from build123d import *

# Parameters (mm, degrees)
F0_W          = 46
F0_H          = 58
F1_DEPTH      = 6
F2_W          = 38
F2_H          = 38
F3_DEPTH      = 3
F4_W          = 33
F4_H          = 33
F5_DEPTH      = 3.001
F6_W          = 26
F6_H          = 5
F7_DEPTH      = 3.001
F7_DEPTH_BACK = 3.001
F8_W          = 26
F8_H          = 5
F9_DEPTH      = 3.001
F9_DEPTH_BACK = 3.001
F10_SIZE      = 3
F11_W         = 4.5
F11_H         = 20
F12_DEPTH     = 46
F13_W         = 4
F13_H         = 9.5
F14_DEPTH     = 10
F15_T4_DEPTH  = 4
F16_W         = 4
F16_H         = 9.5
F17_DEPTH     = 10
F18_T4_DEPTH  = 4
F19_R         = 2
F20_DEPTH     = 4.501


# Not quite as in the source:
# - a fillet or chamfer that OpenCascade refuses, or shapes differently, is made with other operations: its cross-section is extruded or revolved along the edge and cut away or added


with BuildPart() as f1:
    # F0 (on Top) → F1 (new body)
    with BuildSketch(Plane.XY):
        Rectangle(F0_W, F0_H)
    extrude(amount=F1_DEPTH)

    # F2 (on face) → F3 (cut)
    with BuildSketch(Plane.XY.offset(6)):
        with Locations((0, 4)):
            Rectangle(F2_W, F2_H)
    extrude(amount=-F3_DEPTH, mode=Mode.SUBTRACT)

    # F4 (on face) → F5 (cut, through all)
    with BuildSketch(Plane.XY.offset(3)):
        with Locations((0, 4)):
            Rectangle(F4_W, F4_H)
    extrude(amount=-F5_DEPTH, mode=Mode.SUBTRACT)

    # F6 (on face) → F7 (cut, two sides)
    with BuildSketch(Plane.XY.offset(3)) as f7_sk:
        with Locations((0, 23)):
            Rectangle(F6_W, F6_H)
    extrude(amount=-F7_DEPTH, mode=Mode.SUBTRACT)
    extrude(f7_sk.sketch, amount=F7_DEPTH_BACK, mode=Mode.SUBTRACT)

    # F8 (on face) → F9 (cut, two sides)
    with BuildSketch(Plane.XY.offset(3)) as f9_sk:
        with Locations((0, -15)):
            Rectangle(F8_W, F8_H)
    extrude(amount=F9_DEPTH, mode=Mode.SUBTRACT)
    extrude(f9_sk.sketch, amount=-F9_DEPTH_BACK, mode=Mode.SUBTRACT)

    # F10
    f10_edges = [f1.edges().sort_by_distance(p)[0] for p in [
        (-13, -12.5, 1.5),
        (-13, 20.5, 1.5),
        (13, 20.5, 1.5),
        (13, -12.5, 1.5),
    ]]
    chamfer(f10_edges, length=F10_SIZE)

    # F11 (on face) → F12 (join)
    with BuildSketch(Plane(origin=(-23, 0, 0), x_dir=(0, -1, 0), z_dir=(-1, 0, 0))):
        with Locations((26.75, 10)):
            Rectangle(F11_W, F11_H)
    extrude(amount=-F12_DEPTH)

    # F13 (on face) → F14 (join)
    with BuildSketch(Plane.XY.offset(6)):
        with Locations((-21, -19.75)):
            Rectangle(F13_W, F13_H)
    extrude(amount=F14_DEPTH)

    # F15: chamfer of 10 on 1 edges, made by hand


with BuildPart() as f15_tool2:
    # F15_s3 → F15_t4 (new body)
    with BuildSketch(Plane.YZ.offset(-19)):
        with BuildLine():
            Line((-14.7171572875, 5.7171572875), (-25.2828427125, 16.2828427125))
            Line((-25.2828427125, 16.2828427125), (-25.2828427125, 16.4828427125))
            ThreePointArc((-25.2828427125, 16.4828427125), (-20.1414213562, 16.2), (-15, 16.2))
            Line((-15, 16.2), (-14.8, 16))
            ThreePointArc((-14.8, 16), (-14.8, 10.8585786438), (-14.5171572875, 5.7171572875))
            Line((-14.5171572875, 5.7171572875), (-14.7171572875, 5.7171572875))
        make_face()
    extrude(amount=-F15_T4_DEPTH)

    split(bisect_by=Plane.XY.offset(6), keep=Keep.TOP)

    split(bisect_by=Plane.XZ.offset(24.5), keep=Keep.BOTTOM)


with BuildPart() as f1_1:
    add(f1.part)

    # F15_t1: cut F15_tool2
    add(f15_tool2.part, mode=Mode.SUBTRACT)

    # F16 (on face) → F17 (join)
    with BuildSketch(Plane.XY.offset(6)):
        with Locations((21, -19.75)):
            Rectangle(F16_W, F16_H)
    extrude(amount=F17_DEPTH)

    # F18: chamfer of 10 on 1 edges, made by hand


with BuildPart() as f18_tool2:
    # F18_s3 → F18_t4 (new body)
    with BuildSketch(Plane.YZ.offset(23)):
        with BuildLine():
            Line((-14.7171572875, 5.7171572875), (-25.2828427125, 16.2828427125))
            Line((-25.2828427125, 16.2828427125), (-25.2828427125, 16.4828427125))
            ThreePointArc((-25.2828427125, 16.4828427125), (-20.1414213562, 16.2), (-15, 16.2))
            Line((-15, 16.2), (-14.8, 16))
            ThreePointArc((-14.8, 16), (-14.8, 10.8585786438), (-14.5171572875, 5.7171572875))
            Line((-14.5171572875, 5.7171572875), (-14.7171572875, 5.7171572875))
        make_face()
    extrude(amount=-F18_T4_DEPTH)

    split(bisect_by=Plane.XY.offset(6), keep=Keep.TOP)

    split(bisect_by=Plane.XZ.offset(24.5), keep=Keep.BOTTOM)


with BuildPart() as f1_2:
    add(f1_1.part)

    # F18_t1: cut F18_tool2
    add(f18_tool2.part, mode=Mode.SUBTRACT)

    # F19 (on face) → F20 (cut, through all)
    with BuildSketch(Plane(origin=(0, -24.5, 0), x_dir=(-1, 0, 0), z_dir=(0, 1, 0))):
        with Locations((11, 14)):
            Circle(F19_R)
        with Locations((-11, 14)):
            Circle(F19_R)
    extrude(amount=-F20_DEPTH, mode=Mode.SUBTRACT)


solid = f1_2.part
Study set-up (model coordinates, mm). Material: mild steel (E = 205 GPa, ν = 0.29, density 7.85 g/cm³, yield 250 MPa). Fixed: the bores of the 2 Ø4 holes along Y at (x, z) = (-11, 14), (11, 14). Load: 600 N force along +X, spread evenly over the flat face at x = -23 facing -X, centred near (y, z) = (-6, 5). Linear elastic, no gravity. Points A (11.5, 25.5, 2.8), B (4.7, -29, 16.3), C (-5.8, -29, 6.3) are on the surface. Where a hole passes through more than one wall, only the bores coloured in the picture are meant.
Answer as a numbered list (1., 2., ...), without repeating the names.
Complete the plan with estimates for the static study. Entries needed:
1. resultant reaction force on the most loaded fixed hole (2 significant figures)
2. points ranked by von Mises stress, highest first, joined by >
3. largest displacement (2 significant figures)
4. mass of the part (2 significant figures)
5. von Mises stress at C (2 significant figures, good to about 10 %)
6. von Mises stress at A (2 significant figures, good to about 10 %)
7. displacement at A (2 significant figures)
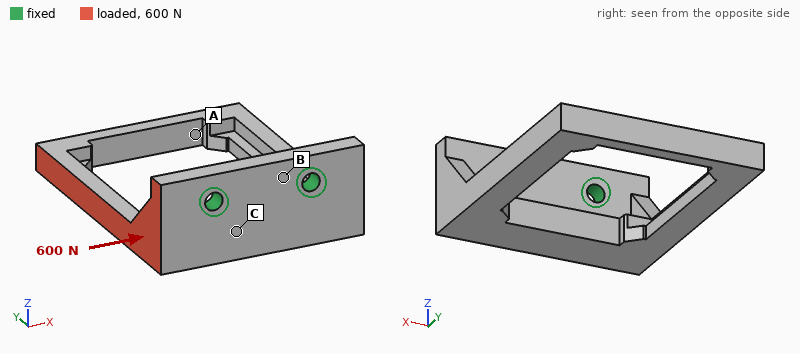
1. 580 N
2. A > C > B
3. 85 µm
4. 81 g
5. 17 MPa
6. 71 MPa
7. 74 µm
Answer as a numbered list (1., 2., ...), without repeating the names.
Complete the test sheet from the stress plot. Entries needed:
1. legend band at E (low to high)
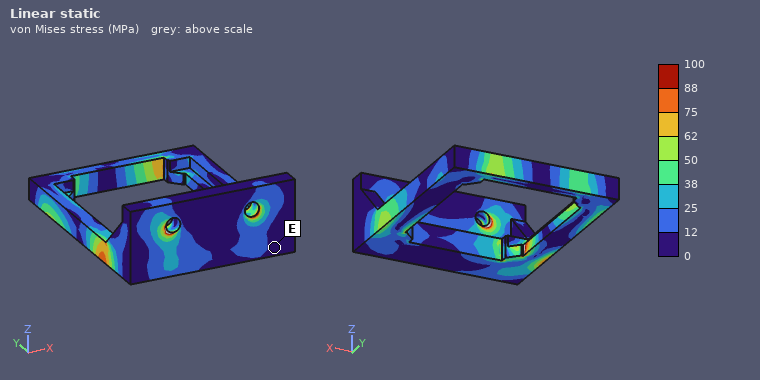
1. 0 to 12 MPa
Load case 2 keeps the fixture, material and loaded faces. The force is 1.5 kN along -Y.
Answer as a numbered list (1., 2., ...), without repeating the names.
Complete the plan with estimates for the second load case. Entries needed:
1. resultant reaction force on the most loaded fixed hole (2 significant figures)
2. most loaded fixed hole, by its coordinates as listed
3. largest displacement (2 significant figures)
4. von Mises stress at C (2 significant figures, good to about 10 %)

1. 1.9 kN
2. (-11, 14)
3. 0.11 mm
4. 70 MPa
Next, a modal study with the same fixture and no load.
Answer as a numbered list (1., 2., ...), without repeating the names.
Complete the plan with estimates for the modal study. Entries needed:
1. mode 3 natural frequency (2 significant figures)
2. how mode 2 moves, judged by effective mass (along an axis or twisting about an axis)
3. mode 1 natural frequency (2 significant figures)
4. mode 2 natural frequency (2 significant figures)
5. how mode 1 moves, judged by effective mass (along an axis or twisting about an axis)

1. 2700 Hz
2. along X
3. 1200 Hz
4. 1900 Hz
5. along Z
